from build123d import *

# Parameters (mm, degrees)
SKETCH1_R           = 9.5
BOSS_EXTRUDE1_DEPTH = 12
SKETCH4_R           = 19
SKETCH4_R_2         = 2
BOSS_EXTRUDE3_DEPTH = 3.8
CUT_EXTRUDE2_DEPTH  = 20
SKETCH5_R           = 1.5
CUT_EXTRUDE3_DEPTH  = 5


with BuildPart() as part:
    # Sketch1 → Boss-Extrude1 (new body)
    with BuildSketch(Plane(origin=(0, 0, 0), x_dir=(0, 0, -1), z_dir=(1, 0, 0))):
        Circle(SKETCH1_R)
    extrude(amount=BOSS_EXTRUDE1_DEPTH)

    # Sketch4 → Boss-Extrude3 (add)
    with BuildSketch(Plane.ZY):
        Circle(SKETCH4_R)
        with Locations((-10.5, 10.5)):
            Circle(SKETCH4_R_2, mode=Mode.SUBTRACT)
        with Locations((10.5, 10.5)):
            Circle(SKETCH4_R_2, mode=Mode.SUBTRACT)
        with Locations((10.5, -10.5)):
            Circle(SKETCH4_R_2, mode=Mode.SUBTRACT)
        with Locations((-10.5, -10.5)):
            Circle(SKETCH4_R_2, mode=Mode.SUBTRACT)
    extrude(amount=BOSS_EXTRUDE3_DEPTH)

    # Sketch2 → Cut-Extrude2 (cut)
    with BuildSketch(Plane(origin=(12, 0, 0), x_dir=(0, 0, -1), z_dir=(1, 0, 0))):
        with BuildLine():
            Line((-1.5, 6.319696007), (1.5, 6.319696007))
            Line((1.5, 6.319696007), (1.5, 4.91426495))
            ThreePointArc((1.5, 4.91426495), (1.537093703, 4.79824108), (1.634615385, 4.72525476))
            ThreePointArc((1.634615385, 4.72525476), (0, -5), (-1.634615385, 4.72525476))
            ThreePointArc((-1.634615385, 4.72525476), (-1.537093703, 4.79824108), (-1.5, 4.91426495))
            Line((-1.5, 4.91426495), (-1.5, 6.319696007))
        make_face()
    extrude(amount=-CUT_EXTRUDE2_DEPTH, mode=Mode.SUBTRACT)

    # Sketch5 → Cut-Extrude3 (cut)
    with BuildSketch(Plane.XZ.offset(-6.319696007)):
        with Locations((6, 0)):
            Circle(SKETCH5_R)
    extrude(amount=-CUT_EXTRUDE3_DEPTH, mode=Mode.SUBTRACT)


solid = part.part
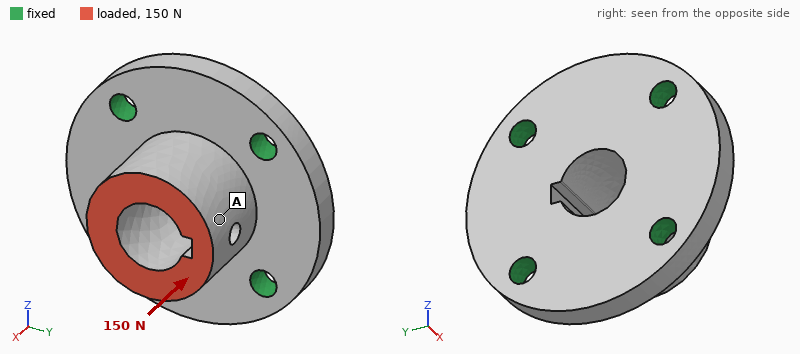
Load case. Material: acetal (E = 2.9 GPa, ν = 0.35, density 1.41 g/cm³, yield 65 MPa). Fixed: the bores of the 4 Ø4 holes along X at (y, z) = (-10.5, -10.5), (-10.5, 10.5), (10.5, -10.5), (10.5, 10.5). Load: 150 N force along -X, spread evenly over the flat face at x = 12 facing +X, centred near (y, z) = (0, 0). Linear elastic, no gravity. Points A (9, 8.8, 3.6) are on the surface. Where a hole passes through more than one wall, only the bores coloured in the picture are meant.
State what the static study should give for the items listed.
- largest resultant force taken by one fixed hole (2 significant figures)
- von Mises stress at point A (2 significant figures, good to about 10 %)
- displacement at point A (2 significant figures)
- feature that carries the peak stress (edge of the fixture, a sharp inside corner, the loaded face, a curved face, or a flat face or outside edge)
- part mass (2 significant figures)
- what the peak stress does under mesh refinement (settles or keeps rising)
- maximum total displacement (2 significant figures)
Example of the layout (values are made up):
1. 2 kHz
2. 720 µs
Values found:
1. 40 N
2. 0.81 MPa
3. 13 µm
4. edge of the fixture
5. 8.7 g
6. keeps rising
7. 14 µm
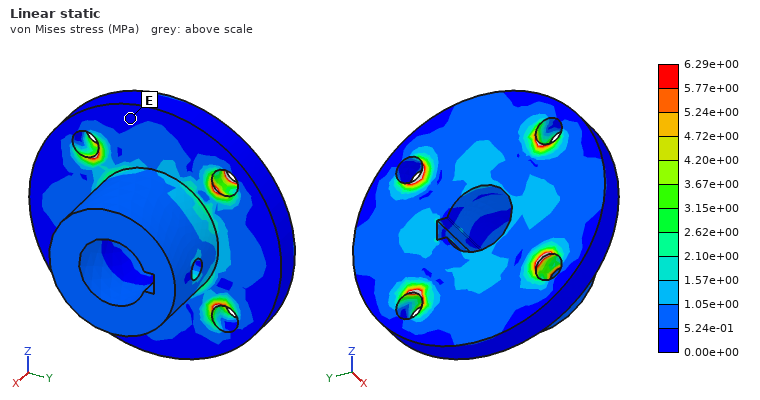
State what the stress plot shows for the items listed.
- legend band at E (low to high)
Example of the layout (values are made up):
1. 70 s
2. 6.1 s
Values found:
1. 0.00e+00 to 5.24e-01 MPa
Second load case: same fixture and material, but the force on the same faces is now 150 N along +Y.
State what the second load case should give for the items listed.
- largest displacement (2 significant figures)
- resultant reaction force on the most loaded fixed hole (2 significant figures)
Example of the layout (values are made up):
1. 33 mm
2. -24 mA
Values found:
1. 56 µm
2. 69 N
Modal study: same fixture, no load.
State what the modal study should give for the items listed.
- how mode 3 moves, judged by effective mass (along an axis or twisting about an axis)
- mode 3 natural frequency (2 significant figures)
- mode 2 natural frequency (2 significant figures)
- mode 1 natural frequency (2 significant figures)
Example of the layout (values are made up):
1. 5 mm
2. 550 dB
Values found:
1. along X
2. 8100 Hz
3. 7000 Hz
4. 6900 Hz
